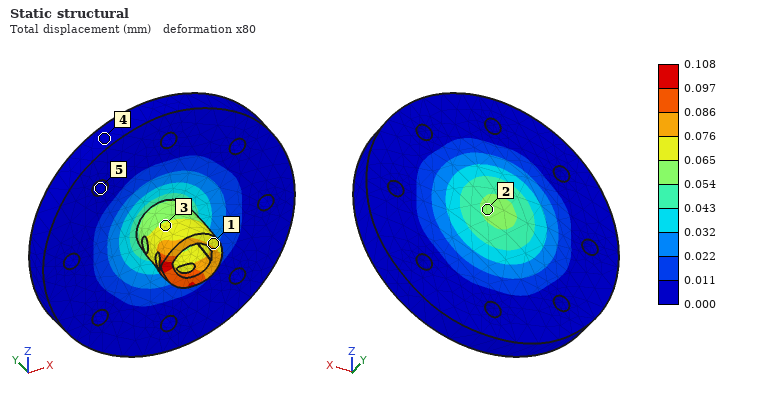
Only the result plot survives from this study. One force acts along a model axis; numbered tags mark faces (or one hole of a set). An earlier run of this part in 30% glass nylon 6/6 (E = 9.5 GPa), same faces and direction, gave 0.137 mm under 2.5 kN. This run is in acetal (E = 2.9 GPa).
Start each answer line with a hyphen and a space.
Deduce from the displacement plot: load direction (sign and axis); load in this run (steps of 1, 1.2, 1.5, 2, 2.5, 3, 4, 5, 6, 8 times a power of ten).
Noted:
- +Y
- 600 N
